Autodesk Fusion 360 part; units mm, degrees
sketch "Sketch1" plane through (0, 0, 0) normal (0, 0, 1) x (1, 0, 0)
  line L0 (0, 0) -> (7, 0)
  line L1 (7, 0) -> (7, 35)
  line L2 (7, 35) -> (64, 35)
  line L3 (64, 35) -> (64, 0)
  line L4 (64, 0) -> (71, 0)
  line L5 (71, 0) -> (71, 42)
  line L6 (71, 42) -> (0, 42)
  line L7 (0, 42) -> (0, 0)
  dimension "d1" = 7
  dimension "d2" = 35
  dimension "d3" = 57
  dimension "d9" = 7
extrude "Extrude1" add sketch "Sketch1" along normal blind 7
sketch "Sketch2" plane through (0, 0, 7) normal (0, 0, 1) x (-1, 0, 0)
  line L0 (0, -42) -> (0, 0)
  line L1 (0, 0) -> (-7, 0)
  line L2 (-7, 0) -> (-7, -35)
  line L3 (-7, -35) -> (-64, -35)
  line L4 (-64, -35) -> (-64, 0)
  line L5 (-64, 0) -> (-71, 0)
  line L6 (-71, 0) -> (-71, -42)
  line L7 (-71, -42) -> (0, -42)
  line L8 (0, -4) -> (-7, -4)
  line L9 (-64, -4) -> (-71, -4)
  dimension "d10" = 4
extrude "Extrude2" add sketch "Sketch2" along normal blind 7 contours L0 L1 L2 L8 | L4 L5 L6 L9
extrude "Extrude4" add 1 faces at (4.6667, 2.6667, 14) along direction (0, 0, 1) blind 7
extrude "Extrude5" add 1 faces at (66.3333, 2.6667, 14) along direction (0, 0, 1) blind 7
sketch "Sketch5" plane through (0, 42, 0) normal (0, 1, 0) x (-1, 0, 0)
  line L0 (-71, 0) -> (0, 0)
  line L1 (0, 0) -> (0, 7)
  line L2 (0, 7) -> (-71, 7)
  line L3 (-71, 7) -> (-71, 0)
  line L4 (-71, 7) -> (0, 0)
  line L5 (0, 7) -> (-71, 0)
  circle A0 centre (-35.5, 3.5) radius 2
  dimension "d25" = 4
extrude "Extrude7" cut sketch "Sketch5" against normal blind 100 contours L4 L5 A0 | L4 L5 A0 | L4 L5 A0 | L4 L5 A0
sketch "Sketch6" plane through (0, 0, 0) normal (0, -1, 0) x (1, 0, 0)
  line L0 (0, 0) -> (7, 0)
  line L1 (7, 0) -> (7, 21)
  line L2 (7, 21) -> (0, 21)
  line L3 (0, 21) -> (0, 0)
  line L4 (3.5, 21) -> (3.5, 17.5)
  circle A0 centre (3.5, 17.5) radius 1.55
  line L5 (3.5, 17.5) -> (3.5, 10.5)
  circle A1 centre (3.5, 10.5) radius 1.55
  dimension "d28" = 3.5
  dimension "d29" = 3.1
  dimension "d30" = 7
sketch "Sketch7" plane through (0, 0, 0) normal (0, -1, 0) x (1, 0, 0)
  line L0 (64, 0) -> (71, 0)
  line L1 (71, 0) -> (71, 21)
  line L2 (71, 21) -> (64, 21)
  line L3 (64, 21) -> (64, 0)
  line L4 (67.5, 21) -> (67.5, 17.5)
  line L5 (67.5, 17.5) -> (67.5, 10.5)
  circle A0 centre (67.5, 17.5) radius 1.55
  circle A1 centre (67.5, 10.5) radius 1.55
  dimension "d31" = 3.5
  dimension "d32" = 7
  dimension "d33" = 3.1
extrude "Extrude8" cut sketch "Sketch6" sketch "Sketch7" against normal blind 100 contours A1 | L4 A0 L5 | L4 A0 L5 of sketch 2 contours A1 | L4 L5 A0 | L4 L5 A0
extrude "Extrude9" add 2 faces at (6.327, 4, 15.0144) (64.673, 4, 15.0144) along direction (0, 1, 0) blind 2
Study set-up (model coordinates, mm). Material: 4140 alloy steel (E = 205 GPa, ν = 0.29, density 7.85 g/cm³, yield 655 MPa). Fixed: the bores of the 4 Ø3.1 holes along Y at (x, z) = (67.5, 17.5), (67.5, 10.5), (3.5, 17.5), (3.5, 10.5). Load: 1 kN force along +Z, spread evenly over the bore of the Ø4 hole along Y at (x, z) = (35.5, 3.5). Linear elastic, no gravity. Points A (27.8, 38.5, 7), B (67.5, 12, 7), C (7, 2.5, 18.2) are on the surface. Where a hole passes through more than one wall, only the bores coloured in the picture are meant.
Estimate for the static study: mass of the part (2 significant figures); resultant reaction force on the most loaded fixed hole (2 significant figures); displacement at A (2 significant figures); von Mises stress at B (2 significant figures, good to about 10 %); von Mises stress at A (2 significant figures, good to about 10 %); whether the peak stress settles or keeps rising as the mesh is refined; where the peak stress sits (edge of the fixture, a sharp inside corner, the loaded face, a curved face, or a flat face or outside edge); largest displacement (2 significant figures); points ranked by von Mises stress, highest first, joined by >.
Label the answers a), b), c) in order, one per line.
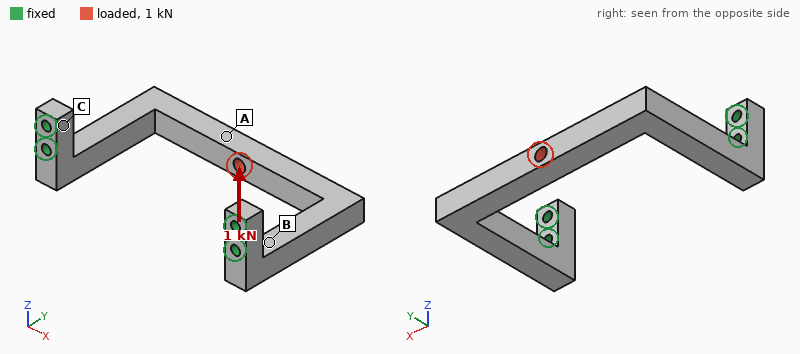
a) 61 g
b) 510 N
c) 0.39 mm
d) 240 MPa
e) 160 MPa
f) keeps rising
g) edge of the fixture
h) 0.44 mm
i) B > A > C
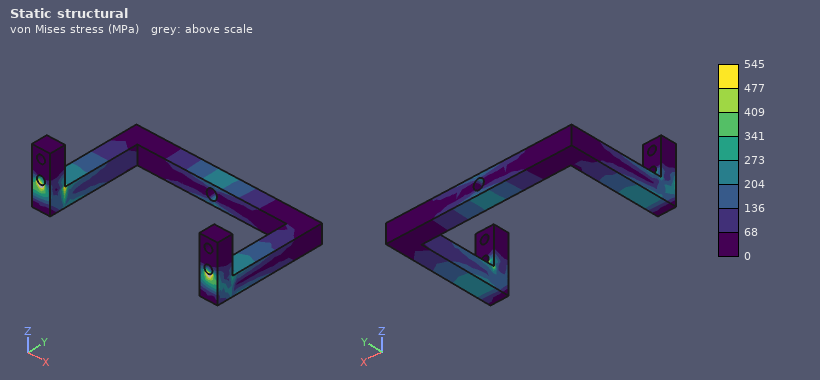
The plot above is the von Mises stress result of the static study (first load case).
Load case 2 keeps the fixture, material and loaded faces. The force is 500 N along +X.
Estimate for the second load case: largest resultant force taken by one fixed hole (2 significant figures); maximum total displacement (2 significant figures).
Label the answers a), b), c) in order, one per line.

a) 340 N
b) 60 µm
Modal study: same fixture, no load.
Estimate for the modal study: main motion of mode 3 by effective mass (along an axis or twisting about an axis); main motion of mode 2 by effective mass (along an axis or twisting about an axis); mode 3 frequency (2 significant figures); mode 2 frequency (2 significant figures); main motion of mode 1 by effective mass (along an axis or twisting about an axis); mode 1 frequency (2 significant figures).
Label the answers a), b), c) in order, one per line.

a) twisting about Y
b) along X
c) 3000 Hz
d) 2600 Hz
e) along Z
f) 1600 Hz
